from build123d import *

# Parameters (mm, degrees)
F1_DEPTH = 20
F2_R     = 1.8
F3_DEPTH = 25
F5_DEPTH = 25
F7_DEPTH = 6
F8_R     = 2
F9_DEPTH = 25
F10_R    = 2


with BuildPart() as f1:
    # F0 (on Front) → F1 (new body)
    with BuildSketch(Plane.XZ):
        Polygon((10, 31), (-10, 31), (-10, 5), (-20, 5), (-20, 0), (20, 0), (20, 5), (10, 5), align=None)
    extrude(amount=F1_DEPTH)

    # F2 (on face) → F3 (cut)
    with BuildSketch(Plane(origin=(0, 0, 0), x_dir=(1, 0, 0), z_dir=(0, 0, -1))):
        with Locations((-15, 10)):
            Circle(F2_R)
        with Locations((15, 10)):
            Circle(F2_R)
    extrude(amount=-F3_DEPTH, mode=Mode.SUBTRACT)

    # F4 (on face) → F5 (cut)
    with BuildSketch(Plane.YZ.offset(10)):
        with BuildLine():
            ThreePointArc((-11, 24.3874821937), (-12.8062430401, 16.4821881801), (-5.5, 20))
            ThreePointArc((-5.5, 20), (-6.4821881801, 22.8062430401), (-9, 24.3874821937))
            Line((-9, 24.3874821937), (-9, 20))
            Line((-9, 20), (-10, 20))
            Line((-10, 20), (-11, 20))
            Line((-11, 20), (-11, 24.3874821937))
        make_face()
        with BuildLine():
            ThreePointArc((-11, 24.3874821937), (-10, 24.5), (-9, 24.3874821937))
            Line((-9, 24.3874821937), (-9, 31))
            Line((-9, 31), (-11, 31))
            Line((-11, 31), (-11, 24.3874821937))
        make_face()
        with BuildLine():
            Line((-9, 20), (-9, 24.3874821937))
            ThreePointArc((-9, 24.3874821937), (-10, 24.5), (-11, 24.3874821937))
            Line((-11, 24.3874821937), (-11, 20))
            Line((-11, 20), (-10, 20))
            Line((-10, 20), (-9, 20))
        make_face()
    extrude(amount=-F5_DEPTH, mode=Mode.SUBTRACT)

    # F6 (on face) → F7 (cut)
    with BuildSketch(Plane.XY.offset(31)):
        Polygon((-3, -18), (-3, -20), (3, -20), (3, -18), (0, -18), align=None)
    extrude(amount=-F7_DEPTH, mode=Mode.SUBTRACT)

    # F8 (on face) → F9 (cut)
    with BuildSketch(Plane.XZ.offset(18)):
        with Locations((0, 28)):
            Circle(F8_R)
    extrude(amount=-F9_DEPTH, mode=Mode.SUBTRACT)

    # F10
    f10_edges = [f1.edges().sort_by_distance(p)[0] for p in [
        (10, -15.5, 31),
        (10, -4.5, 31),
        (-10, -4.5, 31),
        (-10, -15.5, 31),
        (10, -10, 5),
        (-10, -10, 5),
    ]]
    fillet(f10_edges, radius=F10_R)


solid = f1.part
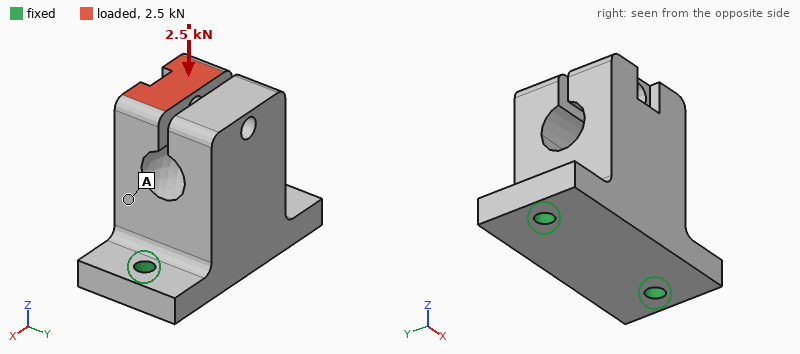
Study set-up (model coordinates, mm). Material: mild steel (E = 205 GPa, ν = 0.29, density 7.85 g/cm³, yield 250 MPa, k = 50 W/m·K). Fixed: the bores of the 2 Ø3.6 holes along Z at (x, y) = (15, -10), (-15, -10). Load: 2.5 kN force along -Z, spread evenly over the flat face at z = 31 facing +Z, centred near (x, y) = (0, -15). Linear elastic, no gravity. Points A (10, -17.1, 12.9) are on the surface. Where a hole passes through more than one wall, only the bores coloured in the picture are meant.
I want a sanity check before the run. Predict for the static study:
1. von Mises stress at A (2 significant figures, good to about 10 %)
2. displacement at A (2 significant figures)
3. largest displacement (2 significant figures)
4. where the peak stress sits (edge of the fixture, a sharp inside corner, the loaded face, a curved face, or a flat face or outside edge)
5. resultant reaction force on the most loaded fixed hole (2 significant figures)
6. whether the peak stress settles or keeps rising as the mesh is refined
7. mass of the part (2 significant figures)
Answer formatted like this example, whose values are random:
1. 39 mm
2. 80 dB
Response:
1. 22 MPa
2. 11 µm
3. 20 µm
4. edge of the fixture
5. 1.4 kN
6. keeps rising
7. 98 g
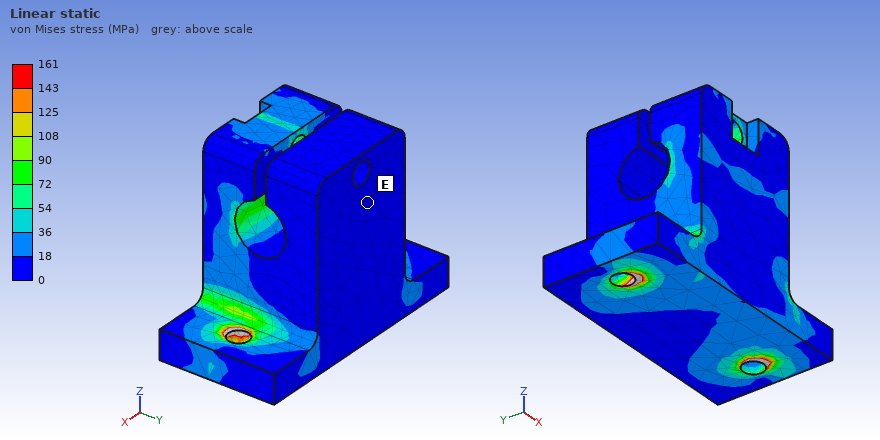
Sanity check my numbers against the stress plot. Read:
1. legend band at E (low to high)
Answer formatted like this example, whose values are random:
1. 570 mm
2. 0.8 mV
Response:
1. 0 to 18 MPa
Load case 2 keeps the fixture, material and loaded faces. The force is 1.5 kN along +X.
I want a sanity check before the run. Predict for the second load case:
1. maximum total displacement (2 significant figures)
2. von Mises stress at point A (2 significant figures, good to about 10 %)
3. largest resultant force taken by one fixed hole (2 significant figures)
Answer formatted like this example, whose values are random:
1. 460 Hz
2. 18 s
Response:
1. 22 µm
2. 56 MPa
3. 1.8 kN
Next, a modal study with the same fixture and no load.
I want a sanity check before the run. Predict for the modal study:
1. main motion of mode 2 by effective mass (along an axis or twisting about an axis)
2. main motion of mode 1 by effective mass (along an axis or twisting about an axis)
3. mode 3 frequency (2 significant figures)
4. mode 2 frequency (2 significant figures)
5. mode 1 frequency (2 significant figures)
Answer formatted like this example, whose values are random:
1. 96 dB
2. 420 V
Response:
1. along X
2. along Y
3. 13 kHz
4. 11 kHz
5. 4400 Hz
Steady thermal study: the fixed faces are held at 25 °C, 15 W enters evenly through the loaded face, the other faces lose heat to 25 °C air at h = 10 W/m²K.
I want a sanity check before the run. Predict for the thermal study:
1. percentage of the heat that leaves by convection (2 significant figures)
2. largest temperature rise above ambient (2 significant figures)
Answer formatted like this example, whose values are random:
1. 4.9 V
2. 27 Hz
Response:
1. 6.2 %
2. 70 K
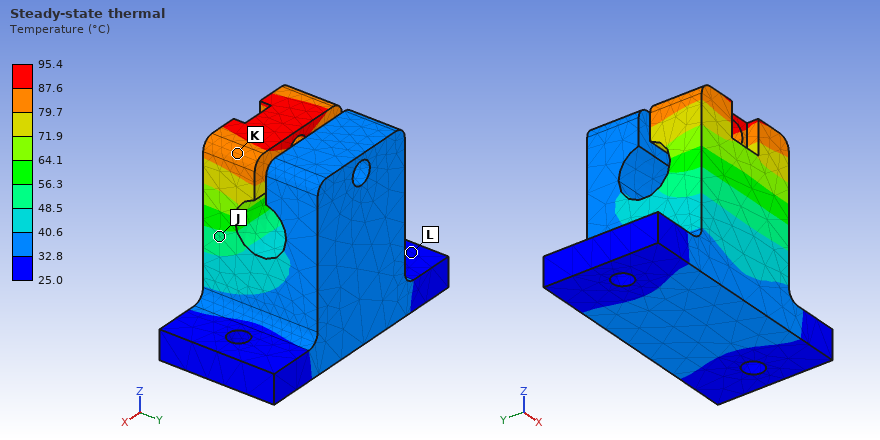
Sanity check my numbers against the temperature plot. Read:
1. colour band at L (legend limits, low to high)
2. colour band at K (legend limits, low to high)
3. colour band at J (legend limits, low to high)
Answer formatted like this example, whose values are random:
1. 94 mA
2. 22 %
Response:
1. 25.0 to 32.8 °C
2. 79.7 to 87.6 °C
3. 48.5 to 56.3 °C
